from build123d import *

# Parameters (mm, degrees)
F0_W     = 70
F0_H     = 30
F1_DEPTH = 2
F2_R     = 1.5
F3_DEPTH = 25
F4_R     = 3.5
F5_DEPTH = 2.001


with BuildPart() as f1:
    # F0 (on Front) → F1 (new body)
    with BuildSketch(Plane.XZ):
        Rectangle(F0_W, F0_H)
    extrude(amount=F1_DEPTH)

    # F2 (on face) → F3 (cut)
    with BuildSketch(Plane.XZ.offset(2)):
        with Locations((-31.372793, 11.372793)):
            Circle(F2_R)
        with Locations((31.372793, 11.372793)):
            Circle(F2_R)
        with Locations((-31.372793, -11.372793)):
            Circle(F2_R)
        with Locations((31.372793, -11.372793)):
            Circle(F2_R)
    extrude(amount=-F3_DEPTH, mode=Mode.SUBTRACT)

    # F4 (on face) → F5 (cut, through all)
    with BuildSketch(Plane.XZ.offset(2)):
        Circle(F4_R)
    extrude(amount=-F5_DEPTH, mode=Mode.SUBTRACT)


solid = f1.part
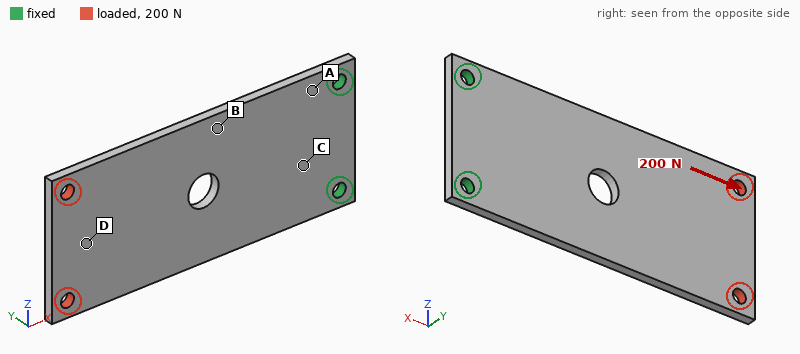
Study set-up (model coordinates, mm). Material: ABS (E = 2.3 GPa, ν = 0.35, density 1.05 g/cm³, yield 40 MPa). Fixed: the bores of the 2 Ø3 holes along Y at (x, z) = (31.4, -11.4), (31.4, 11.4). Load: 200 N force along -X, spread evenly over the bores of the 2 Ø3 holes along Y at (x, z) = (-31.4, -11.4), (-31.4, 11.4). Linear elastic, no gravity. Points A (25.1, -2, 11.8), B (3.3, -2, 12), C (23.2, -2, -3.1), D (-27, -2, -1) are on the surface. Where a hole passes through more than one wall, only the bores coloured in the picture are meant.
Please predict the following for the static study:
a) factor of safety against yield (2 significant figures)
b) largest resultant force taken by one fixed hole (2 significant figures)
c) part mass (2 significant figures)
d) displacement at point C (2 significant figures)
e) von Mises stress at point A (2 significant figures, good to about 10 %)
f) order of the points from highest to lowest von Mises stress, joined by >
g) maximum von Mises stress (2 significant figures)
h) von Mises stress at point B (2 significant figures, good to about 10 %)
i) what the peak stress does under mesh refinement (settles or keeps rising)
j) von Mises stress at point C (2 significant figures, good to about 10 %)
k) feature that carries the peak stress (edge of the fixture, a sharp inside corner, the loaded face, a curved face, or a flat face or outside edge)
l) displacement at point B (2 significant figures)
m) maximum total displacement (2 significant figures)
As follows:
2.5
100 N
4.3 g
0.024 mm
5.2 MPa
A > B > C > D
16 MPa
3.6 MPa
settles
2.1 MPa
the loaded face
0.052 mm
0.13 mm
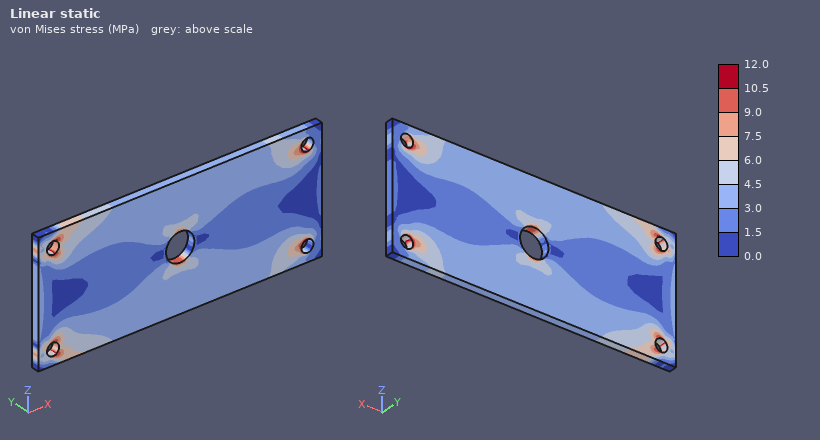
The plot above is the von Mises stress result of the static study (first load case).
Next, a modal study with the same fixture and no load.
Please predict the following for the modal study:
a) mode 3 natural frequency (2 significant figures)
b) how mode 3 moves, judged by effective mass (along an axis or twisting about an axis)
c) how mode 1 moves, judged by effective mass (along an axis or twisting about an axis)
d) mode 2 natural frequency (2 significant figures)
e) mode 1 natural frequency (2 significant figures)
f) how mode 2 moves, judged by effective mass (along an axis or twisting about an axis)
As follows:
670 Hz
along Y
along Y
510 Hz
110 Hz
twisting about X
